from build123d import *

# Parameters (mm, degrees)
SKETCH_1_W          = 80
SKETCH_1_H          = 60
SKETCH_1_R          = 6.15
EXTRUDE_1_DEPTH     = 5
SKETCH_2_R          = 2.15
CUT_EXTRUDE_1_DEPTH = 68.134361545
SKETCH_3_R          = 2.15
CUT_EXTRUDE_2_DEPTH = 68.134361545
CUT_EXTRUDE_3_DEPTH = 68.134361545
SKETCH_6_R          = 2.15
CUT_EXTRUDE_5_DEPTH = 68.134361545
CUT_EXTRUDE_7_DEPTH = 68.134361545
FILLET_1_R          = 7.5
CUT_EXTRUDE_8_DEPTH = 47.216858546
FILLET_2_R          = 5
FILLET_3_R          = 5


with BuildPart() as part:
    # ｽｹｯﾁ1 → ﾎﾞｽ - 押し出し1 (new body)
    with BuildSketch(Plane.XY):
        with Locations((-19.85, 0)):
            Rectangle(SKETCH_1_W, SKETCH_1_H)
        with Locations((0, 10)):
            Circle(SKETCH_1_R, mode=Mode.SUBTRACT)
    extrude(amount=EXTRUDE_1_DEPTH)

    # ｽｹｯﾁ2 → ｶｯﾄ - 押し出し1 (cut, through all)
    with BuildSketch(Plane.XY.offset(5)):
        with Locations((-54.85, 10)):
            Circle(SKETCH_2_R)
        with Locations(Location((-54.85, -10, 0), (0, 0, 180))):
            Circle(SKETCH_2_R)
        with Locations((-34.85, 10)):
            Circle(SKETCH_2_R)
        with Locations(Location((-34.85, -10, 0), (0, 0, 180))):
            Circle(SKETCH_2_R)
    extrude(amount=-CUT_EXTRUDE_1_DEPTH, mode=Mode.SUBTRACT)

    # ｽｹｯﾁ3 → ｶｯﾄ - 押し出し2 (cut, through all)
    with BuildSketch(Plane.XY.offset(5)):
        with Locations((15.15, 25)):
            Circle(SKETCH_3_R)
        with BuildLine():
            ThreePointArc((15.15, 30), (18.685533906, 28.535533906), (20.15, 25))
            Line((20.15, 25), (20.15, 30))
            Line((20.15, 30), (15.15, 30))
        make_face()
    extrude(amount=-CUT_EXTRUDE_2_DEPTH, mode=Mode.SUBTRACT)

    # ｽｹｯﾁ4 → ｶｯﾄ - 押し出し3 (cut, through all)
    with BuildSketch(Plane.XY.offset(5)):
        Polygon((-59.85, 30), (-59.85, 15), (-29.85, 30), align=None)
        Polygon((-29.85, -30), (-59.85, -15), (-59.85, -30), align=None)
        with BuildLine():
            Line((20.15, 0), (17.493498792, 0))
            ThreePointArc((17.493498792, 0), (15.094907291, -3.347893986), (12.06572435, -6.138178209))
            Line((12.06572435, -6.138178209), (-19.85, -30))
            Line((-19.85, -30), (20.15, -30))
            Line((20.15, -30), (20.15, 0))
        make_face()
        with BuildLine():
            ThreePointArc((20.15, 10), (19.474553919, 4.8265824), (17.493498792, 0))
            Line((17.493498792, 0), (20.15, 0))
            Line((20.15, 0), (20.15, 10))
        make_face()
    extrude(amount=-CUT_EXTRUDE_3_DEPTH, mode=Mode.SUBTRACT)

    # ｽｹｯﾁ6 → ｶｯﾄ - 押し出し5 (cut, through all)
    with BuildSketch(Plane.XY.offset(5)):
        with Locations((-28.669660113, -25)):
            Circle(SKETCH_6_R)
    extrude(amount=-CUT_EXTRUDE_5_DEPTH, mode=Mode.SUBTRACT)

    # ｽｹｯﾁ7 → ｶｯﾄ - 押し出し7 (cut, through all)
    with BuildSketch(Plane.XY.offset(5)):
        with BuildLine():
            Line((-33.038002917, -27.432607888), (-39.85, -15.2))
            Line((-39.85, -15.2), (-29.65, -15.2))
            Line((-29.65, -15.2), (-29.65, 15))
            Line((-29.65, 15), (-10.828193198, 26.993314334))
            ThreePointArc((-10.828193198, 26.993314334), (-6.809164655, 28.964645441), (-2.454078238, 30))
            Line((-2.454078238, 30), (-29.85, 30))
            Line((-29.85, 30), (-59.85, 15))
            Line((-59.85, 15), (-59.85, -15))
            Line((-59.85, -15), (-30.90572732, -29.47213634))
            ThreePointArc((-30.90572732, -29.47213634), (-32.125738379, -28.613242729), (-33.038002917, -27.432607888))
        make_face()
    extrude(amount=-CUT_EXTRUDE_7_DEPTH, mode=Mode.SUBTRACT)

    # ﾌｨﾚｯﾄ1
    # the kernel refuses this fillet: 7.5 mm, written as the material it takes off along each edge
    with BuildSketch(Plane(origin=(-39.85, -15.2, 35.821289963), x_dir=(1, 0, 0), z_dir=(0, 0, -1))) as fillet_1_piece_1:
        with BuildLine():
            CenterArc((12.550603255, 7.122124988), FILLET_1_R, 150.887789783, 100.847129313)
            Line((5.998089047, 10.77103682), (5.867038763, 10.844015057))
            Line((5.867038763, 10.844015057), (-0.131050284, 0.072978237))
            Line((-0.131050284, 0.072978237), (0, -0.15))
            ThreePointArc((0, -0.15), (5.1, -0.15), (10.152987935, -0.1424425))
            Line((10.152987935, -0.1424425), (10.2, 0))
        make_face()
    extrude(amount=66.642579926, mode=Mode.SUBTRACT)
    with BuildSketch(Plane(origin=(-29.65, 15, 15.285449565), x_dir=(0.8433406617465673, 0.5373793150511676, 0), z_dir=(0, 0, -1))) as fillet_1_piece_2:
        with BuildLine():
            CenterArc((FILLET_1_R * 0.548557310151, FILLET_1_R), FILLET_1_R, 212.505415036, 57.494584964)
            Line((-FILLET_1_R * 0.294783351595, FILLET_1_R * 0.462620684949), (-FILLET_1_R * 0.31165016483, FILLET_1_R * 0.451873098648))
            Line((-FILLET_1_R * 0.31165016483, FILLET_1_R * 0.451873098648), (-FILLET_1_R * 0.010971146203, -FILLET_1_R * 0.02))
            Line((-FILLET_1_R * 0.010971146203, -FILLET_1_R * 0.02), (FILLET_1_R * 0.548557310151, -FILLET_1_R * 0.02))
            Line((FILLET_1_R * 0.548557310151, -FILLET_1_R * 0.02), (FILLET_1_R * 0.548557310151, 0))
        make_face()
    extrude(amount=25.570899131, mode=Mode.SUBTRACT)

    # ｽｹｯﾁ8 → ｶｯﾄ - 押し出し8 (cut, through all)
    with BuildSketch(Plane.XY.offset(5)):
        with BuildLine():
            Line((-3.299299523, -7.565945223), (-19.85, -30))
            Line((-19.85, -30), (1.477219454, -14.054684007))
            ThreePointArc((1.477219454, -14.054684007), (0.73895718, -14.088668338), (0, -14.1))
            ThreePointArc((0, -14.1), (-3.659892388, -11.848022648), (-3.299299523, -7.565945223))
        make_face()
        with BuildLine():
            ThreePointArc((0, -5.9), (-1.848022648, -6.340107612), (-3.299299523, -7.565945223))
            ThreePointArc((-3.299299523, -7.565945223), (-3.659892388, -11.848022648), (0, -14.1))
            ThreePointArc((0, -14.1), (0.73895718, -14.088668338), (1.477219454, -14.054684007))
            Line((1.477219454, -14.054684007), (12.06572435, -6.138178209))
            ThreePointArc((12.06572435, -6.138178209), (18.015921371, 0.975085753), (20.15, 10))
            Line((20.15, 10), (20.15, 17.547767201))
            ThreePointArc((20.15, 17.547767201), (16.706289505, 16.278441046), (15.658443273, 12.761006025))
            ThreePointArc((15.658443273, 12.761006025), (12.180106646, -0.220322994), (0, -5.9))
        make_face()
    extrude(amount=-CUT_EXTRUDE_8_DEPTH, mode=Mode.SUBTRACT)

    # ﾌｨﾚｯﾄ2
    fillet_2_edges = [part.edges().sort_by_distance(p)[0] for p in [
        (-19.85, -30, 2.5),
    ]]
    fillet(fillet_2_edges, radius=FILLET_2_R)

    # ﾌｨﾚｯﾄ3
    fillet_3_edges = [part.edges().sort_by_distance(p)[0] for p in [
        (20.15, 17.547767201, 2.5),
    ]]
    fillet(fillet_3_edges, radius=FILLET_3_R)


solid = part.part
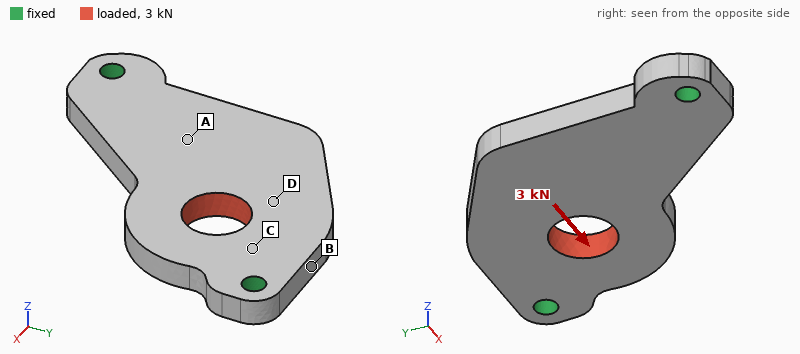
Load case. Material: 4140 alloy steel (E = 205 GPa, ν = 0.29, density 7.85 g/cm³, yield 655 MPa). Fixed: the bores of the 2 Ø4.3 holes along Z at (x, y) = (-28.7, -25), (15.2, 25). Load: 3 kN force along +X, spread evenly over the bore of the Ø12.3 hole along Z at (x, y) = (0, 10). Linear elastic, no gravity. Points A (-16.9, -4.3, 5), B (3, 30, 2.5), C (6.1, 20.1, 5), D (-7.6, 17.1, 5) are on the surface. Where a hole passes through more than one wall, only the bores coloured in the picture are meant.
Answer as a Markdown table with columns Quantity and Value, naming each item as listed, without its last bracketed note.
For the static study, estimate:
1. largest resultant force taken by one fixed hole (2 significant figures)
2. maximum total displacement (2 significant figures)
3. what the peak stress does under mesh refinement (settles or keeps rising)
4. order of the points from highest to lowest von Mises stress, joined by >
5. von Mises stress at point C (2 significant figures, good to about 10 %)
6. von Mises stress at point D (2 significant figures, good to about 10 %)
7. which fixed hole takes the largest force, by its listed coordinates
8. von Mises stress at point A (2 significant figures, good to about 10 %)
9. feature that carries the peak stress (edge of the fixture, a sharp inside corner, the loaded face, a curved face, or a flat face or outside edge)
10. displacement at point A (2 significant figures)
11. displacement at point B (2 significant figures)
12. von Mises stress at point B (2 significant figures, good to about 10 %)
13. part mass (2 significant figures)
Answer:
| Quantity | Value |
|---|---|
| largest resultant force taken by one fixed hole | 2.3 kN |
| maximum total displacement | 7.1 µm |
| what the peak stress does under mesh refinement | keeps rising |
| order of the points from highest to lowest von Mises stress, joined by > | C > B > D > A |
| von Mises stress at point C | 35 MPa |
| von Mises stress at point D | 18 MPa |
| which fixed hole takes the largest force, by its listed coordinates | (15.2, 25) |
| von Mises stress at point A | 8.4 MPa |
| feature that carries the peak stress | edge of the fixture |
| displacement at point A | 5.7 µm |
| displacement at point B | 1.8 µm |
| von Mises stress at point B | 28 MPa |
| part mass | 71 g |
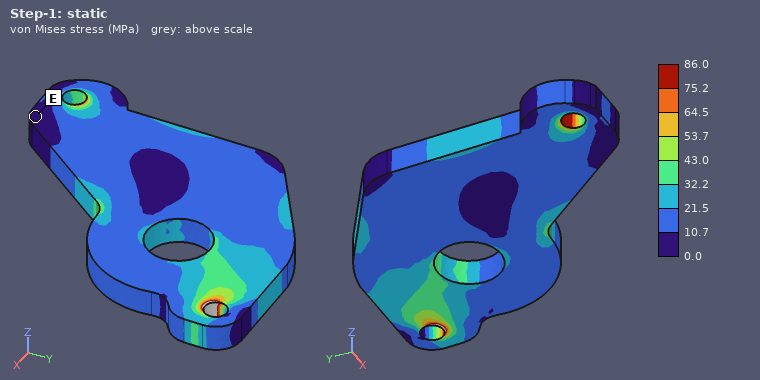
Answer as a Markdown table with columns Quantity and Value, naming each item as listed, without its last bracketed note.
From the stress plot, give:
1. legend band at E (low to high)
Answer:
| Quantity | Value |
|---|---|
| legend band at E | 0.0 to 10.7 MPa |
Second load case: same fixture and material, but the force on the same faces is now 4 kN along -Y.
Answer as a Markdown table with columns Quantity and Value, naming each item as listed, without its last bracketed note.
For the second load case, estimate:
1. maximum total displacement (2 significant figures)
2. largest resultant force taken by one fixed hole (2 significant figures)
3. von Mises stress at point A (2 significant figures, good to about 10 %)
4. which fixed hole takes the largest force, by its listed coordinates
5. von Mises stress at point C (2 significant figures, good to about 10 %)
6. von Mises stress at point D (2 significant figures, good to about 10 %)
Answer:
| Quantity | Value |
|---|---|
| maximum total displacement | 8.4 µm |
| largest resultant force taken by one fixed hole | 2.2 kN |
| von Mises stress at point A | 19 MPa |
| which fixed hole takes the largest force, by its listed coordinates | (15.2, 25) |
| von Mises stress at point C | 26 MPa |
| von Mises stress at point D | 20 MPa |
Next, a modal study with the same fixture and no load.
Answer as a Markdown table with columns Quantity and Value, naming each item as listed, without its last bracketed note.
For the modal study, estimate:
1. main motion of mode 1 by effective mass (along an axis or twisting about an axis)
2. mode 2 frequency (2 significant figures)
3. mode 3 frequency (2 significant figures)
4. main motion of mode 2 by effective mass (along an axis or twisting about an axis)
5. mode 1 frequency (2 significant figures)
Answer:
| Quantity | Value |
|---|---|
| main motion of mode 1 by effective mass | along Z |
| mode 2 frequency | 6200 Hz |
| mode 3 frequency | 12 kHz |
| main motion of mode 2 by effective mass | along Z |
| mode 1 frequency | 3800 Hz |
